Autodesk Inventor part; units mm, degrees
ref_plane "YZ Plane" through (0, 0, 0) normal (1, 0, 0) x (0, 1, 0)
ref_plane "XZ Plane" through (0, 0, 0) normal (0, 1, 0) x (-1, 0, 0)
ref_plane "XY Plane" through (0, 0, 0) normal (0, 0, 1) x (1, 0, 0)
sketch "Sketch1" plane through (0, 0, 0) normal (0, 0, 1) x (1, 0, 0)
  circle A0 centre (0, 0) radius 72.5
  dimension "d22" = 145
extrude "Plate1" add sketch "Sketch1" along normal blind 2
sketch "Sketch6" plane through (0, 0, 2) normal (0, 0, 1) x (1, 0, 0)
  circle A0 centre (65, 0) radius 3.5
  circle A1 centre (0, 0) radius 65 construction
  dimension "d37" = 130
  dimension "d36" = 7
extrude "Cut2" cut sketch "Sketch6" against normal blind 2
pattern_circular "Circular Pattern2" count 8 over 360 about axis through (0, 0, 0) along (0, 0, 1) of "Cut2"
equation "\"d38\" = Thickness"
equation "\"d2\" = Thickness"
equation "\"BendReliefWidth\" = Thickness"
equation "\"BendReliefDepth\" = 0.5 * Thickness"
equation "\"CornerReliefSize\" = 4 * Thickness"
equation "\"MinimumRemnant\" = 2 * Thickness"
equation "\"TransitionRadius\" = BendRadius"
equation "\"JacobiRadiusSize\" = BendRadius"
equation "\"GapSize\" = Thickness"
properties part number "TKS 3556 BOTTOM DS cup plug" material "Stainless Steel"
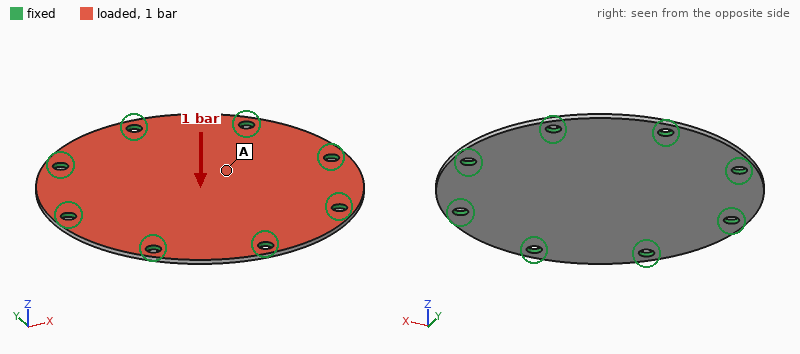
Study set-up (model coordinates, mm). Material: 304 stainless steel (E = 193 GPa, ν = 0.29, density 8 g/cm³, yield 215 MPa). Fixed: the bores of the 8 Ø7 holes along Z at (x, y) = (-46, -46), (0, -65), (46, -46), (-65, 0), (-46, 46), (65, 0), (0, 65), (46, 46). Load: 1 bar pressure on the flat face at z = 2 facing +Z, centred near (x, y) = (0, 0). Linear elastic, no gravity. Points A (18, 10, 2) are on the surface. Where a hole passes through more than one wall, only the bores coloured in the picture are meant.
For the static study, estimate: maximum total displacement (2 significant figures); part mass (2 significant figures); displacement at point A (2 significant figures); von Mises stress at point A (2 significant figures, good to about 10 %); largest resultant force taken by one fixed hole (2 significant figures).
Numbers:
0.21 mm
260 g
0.18 mm
43 MPa
200 N
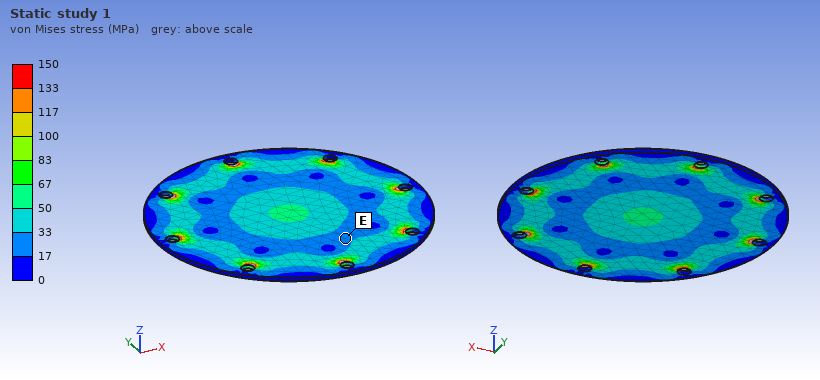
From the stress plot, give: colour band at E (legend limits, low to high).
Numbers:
17 to 33 MPa
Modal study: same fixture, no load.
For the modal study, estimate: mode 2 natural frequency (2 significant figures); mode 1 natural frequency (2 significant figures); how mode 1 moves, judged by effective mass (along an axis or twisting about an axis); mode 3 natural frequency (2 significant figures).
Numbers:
2200 Hz
1100 Hz
along Z
2200 Hz
